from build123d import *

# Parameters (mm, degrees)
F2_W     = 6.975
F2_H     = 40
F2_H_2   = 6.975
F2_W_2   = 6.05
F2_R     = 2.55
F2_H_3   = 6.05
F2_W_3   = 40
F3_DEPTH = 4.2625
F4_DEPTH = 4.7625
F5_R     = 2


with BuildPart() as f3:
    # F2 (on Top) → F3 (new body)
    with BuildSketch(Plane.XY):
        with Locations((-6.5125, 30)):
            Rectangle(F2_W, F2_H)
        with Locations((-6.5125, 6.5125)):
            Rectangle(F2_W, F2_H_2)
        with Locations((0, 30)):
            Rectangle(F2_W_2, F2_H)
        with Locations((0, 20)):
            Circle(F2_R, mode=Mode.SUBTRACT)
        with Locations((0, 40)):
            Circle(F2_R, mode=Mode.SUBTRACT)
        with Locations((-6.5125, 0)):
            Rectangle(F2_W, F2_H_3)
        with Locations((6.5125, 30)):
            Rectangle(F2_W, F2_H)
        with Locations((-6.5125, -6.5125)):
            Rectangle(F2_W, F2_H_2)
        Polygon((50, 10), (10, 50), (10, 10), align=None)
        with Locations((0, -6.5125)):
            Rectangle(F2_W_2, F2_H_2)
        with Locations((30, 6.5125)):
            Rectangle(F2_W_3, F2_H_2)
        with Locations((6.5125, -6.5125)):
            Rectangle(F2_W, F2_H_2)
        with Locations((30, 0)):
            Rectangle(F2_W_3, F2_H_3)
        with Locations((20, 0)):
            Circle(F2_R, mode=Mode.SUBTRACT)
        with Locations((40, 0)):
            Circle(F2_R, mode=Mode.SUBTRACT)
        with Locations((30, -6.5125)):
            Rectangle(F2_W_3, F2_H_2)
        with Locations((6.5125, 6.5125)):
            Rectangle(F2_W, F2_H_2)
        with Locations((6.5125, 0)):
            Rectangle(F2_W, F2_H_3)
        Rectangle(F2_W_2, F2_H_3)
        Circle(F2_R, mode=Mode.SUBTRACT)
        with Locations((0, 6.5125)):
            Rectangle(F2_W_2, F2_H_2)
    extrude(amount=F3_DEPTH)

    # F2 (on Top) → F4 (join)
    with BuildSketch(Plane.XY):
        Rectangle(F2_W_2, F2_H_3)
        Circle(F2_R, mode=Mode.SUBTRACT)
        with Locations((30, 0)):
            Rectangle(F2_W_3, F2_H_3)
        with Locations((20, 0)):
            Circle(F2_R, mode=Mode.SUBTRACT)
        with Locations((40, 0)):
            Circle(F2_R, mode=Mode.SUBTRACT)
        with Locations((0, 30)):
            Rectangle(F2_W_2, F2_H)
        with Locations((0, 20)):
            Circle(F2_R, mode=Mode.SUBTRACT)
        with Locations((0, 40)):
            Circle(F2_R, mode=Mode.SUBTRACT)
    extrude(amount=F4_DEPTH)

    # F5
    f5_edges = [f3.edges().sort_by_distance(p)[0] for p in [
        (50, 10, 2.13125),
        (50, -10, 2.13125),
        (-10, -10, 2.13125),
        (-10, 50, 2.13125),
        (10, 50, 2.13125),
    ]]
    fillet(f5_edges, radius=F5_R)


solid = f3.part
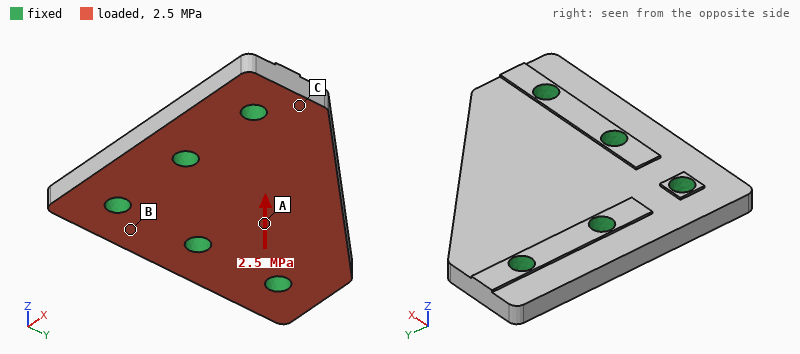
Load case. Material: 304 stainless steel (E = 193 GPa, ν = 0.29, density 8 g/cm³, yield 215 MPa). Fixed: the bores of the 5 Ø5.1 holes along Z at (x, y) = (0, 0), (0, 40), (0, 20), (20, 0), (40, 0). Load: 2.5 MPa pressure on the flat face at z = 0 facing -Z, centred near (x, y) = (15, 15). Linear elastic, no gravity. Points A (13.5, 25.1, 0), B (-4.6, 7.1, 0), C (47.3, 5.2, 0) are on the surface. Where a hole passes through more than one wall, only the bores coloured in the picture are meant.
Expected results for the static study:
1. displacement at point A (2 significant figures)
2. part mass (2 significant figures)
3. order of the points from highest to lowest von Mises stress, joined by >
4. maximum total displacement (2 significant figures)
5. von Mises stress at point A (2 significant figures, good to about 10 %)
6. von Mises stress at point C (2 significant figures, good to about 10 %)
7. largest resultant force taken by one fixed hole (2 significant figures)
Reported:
18 µm
94 g
C > A > B
53 µm
38 MPa
72 MPa
1.6 kN
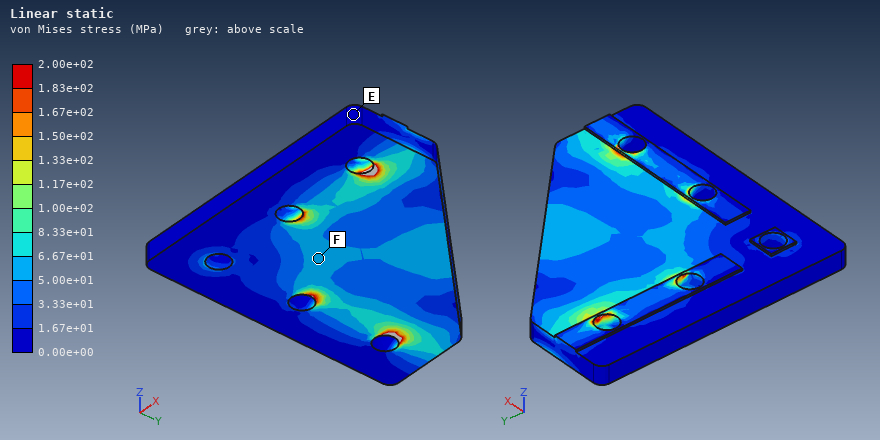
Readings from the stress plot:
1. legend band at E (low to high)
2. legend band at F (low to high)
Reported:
0.00e+00 to 1.67e+01 MPa
5.00e+01 to 6.67e+01 MPa
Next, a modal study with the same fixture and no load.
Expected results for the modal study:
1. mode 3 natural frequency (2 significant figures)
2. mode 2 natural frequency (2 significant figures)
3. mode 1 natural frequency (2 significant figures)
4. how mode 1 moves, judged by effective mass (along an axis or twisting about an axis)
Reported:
22 kHz
16 kHz
8000 Hz
along Z
